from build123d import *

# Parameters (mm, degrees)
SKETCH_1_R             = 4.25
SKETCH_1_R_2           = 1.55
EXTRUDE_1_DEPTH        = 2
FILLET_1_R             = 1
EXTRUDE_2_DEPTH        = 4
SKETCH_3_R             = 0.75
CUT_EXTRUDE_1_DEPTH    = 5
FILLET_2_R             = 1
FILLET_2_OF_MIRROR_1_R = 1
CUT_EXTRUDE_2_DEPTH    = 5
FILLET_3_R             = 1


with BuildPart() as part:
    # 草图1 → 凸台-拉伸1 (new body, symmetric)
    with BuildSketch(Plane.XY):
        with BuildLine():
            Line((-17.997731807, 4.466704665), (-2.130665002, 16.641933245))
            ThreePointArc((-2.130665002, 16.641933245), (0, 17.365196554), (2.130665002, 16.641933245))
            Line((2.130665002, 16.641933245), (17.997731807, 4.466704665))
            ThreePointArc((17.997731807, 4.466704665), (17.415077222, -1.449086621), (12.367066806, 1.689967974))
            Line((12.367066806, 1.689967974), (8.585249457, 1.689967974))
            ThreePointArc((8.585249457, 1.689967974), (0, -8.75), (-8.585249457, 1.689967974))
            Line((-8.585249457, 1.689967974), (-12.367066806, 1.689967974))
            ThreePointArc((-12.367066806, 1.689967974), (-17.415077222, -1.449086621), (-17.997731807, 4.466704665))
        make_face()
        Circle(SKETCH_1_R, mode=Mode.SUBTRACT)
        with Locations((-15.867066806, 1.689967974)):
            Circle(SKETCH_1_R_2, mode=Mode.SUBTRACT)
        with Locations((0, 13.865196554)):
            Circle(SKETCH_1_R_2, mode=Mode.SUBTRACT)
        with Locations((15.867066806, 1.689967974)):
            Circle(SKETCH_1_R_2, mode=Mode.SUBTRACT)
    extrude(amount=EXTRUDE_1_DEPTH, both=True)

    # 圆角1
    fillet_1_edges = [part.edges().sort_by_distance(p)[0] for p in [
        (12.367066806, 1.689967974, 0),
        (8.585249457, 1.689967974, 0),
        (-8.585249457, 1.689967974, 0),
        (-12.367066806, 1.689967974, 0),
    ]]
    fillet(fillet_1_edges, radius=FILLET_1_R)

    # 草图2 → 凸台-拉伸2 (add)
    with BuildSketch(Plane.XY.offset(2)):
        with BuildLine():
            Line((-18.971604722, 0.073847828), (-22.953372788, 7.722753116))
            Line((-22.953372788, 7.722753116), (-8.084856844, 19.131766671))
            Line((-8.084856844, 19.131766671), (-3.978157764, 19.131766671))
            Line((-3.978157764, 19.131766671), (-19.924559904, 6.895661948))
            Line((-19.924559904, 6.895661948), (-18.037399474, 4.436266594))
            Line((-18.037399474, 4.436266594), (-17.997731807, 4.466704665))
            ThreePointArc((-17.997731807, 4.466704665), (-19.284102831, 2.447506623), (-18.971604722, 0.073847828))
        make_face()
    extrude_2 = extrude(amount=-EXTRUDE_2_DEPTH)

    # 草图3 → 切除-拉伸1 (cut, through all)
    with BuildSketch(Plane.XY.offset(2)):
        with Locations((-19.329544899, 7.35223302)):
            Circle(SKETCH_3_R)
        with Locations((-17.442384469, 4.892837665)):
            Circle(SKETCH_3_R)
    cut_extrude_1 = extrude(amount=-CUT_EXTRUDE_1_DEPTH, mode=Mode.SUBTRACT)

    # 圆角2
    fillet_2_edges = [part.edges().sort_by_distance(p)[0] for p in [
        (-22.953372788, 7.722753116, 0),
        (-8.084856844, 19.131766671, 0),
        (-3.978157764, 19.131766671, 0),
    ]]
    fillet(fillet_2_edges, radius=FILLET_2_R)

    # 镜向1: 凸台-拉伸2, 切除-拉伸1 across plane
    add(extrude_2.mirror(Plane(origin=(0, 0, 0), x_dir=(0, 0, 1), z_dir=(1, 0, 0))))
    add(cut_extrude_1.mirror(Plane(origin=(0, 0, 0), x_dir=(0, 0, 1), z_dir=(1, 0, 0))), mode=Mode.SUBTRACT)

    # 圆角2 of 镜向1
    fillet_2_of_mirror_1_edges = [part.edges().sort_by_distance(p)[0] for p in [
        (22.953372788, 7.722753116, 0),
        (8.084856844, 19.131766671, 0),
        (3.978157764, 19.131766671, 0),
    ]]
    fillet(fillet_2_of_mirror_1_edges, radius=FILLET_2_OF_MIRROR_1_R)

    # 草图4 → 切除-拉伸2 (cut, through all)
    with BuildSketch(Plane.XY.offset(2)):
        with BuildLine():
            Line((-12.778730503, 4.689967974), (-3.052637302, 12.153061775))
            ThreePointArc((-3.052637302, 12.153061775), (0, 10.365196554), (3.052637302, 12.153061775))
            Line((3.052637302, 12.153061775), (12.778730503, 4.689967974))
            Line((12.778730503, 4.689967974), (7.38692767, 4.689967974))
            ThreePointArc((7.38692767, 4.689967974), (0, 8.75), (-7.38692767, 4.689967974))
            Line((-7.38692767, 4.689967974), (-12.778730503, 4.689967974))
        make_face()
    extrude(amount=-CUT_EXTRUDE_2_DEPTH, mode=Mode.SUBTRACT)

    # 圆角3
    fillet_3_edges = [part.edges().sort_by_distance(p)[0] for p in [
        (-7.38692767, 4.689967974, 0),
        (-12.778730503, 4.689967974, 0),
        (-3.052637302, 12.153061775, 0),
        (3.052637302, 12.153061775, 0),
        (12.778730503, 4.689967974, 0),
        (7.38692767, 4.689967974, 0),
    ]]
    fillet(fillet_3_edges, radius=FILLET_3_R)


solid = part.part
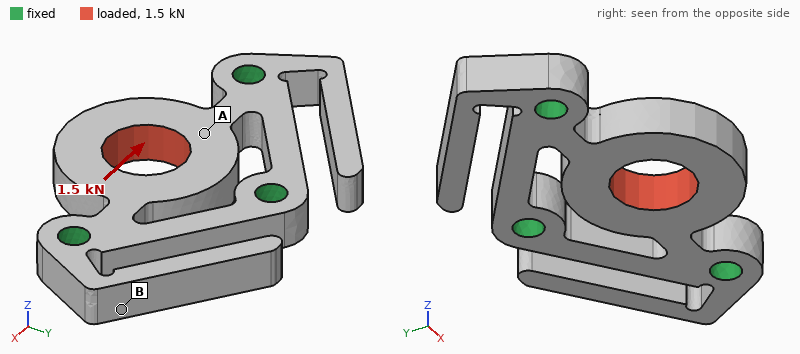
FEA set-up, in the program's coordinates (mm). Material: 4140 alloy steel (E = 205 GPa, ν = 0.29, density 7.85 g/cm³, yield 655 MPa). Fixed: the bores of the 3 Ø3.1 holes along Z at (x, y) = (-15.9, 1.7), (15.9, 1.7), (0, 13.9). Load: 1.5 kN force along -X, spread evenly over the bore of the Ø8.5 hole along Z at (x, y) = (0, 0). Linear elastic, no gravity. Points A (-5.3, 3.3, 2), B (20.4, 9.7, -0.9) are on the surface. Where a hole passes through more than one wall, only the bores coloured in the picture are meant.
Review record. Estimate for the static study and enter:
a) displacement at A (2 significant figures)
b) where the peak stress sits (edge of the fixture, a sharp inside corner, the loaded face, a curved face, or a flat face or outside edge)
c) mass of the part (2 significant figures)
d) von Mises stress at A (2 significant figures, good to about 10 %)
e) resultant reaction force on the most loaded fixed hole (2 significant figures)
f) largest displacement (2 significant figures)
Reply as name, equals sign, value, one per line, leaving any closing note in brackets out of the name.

displacement at A = 2.3 µm
where the peak stress sits = a sharp inside corner
mass of the part = 16 g
von Mises stress at A = 29 MPa
resultant reaction force on the most loaded fixed hole = 710 N
largest displacement = 7.4 µm
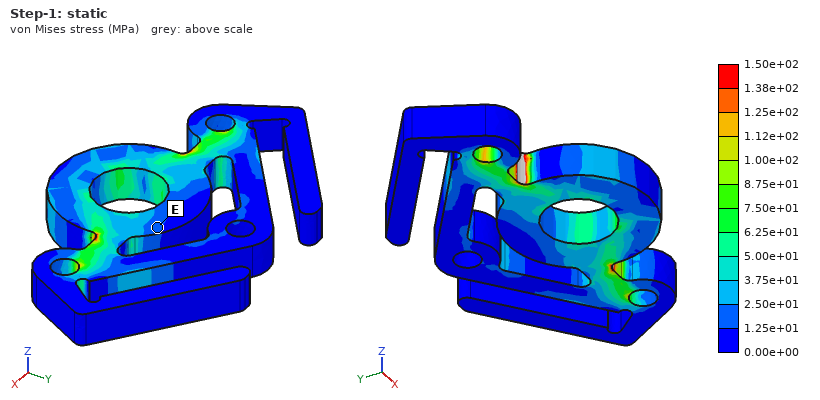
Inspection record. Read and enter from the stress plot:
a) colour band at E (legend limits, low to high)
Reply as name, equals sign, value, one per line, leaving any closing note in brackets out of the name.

colour band at E = 1.25e+01 to 2.50e+01 MPa
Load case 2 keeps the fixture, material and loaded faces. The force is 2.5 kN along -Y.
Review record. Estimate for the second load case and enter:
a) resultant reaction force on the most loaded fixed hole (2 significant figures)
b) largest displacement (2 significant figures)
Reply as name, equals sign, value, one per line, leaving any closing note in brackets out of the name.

resultant reaction force on the most loaded fixed hole = 1.3 kN
largest displacement = 21 µm
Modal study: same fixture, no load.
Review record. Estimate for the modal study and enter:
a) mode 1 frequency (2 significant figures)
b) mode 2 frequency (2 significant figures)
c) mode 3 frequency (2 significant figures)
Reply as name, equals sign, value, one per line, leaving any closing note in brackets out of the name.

mode 1 frequency = 3500 Hz
mode 2 frequency = 3500 Hz
mode 3 frequency = 4500 Hz
